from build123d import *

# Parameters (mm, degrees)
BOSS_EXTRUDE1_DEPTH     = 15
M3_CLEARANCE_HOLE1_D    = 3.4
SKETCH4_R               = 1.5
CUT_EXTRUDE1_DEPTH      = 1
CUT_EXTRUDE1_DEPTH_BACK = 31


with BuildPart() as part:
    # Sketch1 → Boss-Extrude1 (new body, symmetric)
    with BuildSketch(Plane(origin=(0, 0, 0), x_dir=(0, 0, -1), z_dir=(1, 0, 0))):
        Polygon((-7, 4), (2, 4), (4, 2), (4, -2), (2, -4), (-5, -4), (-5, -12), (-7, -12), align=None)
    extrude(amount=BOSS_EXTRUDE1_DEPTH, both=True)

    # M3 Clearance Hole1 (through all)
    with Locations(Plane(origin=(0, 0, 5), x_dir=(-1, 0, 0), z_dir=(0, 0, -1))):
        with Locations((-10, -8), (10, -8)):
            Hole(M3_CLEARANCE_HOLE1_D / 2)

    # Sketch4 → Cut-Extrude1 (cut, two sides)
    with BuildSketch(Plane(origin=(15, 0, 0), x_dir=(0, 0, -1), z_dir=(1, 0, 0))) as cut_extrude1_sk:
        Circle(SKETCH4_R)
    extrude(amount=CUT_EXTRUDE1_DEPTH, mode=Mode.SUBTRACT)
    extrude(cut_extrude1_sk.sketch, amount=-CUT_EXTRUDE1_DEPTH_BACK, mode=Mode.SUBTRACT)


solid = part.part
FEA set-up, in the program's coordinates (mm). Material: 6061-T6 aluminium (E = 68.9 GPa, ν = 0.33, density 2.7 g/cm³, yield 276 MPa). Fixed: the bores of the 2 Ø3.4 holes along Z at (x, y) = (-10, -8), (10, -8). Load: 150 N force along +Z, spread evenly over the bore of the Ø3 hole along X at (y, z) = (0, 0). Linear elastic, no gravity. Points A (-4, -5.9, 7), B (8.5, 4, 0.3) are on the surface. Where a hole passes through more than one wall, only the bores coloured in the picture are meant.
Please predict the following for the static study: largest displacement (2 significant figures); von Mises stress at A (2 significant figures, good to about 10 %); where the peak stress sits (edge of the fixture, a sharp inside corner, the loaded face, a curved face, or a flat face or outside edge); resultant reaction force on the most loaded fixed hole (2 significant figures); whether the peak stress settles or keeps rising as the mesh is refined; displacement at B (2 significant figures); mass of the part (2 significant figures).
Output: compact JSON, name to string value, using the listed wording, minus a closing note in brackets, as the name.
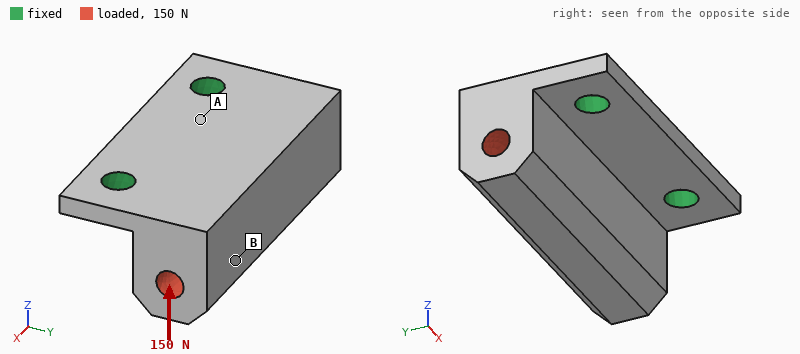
{"largest displacement": "33 µm", "von Mises stress at A": "21 MPa", "where the peak stress sits": "edge of the fixture", "resultant reaction force on the most loaded fixed hole": "75 N", "whether the peak stress settles or keeps rising as the mesh is refined": "keeps rising", "displacement at B": "29 µm", "mass of the part": "7.4 g"}
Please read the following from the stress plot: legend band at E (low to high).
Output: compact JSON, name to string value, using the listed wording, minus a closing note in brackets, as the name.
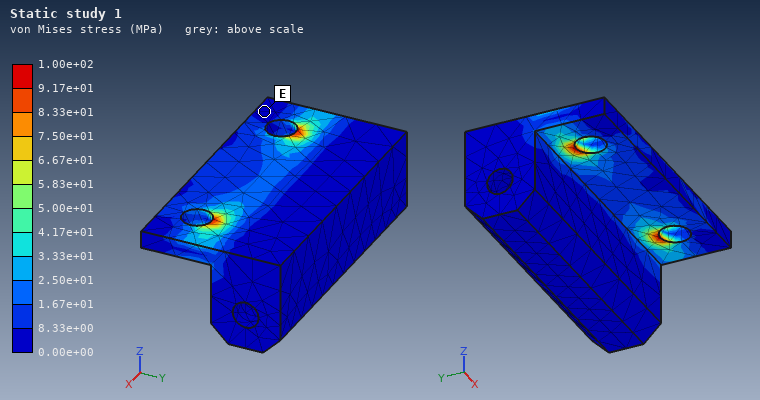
{"legend band at E": "0.00e+00 to 8.33e+00 MPa"}
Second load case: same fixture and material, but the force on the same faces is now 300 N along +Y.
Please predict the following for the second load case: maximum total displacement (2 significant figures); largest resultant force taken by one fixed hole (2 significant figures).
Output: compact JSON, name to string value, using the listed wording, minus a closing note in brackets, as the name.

{"maximum total displacement": "73 µm", "largest resultant force taken by one fixed hole": "150 N"}
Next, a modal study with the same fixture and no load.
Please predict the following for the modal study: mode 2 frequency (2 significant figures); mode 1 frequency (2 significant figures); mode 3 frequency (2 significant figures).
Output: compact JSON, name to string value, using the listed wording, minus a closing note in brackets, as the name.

{"mode 2 frequency": "16 kHz", "mode 1 frequency": "4500 Hz", "mode 3 frequency": "24 kHz"}
